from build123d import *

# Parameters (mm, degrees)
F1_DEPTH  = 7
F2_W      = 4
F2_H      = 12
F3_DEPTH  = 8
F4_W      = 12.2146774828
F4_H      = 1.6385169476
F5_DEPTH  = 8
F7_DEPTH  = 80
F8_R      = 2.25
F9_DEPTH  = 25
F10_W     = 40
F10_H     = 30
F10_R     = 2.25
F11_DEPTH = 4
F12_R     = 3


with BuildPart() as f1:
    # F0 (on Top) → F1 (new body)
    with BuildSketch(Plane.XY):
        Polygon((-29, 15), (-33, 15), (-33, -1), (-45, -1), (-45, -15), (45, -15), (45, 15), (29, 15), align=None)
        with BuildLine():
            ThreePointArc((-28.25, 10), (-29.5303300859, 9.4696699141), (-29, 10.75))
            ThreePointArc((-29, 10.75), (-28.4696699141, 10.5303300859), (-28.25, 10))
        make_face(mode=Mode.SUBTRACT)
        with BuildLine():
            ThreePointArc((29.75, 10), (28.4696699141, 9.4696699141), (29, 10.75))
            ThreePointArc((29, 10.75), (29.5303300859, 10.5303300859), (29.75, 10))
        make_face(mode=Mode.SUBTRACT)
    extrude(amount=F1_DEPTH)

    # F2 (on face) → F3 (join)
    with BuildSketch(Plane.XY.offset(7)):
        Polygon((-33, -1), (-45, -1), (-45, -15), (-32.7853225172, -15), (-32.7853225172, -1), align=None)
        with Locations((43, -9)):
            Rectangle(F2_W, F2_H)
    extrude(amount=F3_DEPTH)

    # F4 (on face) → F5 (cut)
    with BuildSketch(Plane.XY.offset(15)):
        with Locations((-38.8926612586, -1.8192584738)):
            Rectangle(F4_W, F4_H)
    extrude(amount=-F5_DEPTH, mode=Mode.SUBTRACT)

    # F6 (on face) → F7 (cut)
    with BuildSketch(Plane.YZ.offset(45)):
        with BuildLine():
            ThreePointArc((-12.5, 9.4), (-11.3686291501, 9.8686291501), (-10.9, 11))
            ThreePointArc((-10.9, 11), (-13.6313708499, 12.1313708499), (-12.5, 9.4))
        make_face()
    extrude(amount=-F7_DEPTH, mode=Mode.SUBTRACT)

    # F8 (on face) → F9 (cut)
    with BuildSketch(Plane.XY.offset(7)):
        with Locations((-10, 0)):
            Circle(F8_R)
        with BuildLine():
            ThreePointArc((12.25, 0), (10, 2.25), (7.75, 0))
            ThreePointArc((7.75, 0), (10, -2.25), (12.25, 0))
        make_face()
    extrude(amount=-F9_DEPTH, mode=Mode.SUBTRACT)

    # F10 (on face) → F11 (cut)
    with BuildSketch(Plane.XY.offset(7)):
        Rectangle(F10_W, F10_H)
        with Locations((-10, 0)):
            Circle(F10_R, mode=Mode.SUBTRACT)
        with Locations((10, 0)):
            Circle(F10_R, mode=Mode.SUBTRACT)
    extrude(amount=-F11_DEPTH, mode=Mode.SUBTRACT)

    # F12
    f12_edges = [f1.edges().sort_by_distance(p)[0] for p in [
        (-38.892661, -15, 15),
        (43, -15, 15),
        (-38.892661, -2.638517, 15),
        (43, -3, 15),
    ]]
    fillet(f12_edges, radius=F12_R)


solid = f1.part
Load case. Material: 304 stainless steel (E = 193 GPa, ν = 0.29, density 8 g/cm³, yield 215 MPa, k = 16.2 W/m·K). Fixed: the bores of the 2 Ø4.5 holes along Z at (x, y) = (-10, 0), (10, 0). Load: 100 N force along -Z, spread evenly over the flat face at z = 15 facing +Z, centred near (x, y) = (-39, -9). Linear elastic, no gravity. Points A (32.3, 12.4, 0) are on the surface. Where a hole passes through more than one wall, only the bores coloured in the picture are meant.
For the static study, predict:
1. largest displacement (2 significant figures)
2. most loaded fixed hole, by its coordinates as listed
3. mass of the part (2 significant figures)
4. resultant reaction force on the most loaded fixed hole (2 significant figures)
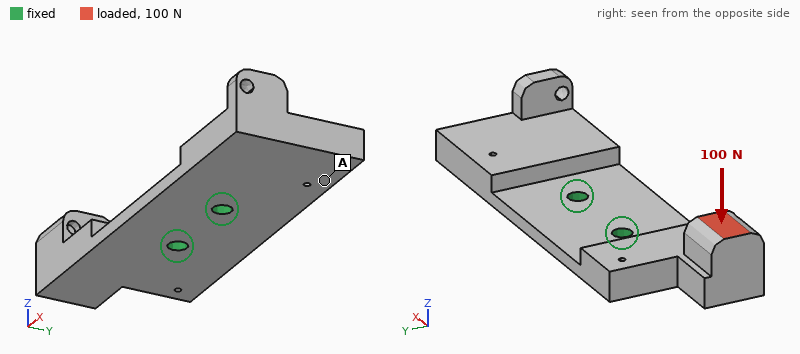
75 µm
(-10, 0)
110 g
140 N
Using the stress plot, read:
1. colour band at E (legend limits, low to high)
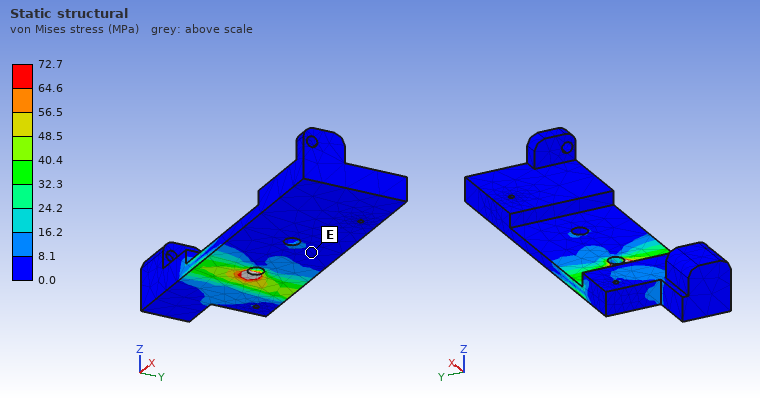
0.0 to 8.1 MPa
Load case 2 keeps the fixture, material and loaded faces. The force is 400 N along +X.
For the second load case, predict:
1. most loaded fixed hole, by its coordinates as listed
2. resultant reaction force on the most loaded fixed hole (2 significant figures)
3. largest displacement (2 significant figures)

(-10, 0)
350 N
0.17 mm
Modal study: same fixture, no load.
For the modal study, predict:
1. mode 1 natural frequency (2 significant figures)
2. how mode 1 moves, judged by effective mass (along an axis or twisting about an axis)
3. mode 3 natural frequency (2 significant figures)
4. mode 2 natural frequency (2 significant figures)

1300 Hz
along Z
3700 Hz
1400 Hz
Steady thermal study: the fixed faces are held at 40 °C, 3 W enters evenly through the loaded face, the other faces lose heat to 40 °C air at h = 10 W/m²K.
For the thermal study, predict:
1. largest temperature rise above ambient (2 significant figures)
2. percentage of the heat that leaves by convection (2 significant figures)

57 K
28 %
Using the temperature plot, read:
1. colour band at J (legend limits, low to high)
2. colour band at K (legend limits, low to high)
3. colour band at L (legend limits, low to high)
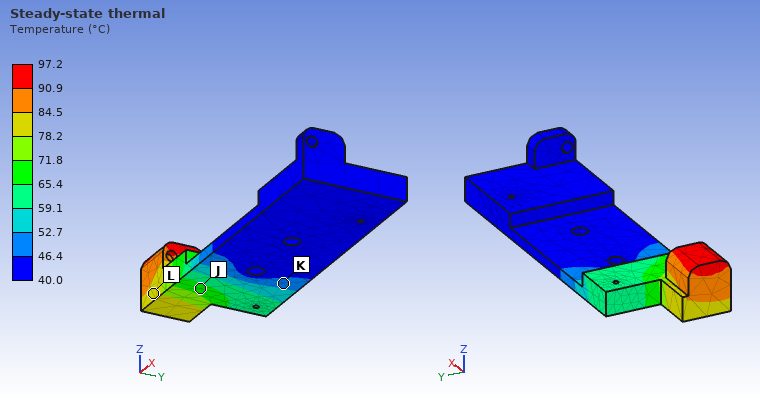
65.4 to 71.8 °C
46.4 to 52.7 °C
78.2 to 84.5 °C
